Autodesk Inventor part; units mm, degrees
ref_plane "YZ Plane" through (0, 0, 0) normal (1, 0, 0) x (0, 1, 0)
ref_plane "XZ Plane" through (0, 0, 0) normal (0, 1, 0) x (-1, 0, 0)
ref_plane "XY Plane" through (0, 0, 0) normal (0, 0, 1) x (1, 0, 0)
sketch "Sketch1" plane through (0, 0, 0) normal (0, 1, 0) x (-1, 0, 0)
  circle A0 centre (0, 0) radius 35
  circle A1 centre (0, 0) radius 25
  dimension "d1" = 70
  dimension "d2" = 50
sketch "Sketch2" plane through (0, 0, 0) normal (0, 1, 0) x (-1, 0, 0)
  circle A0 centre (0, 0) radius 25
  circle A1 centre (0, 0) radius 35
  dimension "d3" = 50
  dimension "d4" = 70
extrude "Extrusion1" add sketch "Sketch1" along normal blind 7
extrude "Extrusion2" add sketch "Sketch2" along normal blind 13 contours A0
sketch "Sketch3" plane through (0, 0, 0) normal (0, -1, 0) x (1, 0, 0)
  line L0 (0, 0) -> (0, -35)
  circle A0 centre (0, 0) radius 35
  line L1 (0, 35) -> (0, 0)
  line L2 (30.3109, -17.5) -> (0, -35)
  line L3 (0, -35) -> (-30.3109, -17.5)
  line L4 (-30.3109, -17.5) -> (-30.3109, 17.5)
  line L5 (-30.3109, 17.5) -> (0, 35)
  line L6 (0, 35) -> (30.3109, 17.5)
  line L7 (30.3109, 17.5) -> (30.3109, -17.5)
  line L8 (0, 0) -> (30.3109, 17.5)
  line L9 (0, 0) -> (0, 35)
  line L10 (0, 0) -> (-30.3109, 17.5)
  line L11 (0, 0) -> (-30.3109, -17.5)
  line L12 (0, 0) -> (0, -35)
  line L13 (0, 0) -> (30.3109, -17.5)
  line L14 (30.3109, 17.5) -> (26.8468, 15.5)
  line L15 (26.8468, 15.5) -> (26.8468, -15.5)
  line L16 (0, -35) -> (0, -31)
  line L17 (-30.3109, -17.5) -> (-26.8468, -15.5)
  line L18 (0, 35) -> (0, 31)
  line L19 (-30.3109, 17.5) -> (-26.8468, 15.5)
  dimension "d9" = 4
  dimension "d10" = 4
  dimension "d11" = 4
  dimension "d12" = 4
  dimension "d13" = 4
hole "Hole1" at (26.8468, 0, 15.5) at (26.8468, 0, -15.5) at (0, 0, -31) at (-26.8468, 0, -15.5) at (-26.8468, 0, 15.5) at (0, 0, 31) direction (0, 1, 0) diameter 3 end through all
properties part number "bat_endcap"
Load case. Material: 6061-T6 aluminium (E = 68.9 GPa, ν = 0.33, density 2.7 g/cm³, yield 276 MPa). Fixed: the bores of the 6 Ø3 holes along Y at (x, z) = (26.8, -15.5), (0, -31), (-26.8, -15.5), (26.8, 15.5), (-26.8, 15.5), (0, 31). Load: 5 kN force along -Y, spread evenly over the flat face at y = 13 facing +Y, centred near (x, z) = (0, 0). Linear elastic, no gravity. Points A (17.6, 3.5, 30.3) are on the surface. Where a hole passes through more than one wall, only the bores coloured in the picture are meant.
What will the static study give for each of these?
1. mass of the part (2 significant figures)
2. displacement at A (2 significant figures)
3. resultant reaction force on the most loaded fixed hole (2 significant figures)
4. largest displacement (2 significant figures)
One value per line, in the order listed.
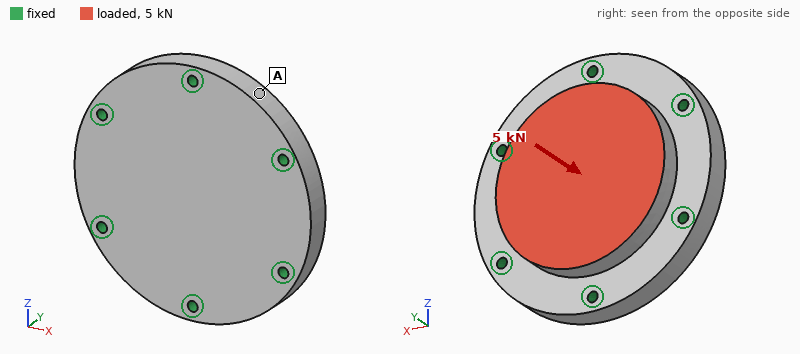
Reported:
100 g
1.7 µm
920 N
10 µm
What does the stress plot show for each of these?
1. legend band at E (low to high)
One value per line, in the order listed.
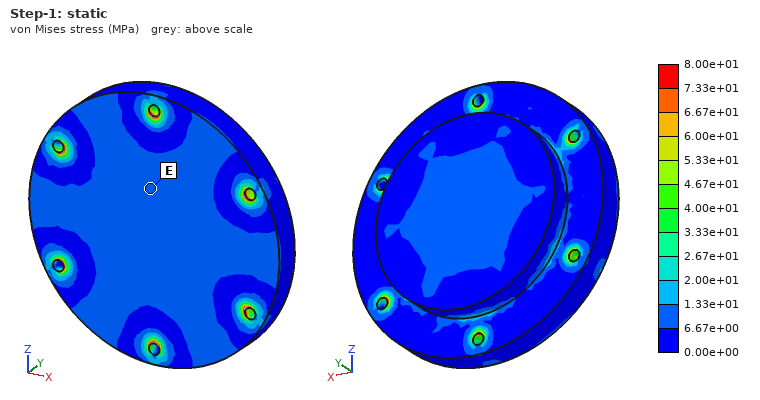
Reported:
6.67e+00 to 1.33e+01 MPa
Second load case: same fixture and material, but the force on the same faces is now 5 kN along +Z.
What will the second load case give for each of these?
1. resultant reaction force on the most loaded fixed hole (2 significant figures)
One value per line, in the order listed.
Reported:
1.2 kN
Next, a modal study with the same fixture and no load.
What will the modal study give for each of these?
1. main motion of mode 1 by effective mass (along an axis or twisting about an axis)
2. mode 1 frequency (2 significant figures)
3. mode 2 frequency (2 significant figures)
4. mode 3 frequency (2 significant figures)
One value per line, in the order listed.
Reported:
along Y
15 kHz
23 kHz
23 kHz
